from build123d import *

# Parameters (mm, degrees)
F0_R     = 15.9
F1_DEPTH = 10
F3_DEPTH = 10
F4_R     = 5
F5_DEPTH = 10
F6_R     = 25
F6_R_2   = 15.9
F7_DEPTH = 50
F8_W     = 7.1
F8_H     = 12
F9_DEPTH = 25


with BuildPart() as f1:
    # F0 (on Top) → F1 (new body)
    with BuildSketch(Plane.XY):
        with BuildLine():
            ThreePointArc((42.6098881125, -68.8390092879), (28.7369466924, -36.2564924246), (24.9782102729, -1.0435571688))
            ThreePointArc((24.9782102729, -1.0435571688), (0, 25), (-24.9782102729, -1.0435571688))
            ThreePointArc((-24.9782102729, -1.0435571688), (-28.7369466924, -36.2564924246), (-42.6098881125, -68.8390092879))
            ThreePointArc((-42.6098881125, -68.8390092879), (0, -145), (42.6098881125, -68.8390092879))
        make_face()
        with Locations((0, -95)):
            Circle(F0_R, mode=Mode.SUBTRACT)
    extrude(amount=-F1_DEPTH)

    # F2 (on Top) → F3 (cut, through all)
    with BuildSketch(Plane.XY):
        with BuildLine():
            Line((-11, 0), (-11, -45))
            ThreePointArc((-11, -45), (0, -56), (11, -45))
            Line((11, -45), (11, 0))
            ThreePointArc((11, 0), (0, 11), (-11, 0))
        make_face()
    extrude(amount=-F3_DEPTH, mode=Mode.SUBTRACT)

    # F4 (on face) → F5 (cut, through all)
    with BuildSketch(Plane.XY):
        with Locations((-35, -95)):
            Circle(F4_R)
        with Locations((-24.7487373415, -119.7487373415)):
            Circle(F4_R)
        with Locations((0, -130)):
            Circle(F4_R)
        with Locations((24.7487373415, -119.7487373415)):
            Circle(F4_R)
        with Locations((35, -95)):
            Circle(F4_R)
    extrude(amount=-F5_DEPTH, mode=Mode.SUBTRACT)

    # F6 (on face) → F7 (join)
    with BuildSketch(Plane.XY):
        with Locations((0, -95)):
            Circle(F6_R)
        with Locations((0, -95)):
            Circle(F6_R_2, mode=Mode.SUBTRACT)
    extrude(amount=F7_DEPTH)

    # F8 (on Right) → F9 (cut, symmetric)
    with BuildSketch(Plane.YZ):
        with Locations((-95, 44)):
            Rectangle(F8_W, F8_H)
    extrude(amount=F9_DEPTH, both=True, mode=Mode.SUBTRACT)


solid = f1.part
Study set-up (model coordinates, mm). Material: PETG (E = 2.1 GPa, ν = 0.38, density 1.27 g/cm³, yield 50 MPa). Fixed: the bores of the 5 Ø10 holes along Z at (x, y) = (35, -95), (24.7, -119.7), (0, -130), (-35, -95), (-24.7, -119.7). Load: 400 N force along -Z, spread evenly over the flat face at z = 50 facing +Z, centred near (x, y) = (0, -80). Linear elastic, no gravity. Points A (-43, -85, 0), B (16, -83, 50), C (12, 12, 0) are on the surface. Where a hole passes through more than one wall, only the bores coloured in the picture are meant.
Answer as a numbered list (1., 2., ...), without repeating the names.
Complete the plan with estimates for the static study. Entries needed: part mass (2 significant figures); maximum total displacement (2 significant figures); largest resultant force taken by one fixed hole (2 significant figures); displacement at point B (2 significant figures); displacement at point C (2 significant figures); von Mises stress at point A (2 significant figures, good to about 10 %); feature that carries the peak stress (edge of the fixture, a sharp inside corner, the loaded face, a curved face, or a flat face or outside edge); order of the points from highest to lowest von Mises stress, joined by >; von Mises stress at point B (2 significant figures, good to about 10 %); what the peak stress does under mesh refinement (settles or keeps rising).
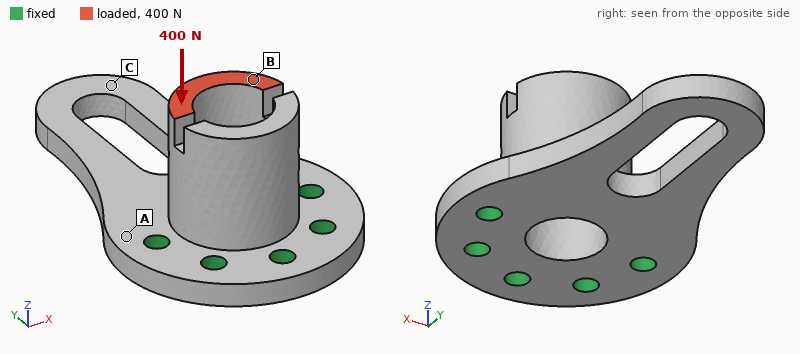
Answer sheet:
1. 190 g
2. 0.28 mm
3. 250 N
4. 0.13 mm
5. 0.25 mm
6. 1.2 MPa
7. edge of the fixture
8. A > B > C
9. 0.76 MPa
10. keeps rising
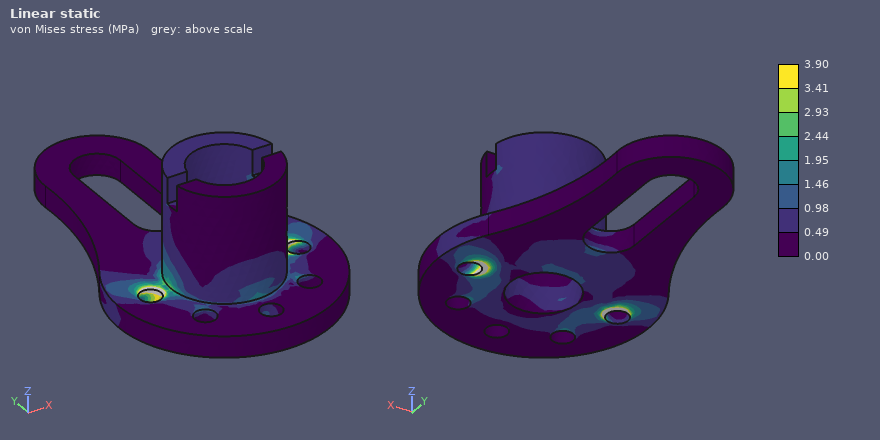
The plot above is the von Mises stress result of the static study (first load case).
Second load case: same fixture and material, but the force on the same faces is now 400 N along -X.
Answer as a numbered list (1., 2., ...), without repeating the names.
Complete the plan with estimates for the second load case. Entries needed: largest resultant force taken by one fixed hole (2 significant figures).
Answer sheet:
1. 340 N
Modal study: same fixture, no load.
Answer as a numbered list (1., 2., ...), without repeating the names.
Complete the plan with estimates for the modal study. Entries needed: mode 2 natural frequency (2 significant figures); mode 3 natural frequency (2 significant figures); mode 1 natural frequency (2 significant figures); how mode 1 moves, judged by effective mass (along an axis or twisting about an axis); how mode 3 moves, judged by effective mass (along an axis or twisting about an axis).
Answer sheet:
1. 730 Hz
2. 890 Hz
3. 240 Hz
4. along Z
5. along X
